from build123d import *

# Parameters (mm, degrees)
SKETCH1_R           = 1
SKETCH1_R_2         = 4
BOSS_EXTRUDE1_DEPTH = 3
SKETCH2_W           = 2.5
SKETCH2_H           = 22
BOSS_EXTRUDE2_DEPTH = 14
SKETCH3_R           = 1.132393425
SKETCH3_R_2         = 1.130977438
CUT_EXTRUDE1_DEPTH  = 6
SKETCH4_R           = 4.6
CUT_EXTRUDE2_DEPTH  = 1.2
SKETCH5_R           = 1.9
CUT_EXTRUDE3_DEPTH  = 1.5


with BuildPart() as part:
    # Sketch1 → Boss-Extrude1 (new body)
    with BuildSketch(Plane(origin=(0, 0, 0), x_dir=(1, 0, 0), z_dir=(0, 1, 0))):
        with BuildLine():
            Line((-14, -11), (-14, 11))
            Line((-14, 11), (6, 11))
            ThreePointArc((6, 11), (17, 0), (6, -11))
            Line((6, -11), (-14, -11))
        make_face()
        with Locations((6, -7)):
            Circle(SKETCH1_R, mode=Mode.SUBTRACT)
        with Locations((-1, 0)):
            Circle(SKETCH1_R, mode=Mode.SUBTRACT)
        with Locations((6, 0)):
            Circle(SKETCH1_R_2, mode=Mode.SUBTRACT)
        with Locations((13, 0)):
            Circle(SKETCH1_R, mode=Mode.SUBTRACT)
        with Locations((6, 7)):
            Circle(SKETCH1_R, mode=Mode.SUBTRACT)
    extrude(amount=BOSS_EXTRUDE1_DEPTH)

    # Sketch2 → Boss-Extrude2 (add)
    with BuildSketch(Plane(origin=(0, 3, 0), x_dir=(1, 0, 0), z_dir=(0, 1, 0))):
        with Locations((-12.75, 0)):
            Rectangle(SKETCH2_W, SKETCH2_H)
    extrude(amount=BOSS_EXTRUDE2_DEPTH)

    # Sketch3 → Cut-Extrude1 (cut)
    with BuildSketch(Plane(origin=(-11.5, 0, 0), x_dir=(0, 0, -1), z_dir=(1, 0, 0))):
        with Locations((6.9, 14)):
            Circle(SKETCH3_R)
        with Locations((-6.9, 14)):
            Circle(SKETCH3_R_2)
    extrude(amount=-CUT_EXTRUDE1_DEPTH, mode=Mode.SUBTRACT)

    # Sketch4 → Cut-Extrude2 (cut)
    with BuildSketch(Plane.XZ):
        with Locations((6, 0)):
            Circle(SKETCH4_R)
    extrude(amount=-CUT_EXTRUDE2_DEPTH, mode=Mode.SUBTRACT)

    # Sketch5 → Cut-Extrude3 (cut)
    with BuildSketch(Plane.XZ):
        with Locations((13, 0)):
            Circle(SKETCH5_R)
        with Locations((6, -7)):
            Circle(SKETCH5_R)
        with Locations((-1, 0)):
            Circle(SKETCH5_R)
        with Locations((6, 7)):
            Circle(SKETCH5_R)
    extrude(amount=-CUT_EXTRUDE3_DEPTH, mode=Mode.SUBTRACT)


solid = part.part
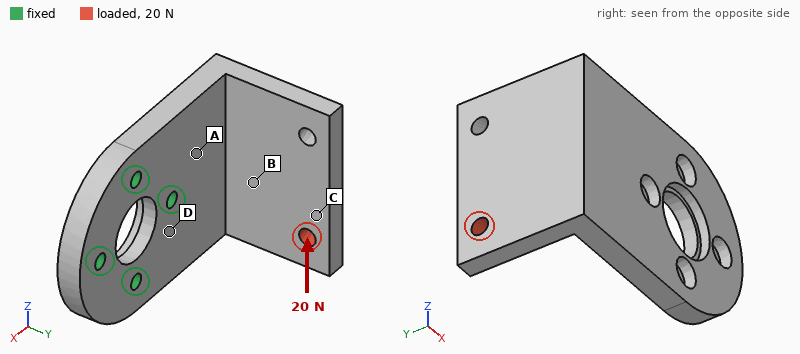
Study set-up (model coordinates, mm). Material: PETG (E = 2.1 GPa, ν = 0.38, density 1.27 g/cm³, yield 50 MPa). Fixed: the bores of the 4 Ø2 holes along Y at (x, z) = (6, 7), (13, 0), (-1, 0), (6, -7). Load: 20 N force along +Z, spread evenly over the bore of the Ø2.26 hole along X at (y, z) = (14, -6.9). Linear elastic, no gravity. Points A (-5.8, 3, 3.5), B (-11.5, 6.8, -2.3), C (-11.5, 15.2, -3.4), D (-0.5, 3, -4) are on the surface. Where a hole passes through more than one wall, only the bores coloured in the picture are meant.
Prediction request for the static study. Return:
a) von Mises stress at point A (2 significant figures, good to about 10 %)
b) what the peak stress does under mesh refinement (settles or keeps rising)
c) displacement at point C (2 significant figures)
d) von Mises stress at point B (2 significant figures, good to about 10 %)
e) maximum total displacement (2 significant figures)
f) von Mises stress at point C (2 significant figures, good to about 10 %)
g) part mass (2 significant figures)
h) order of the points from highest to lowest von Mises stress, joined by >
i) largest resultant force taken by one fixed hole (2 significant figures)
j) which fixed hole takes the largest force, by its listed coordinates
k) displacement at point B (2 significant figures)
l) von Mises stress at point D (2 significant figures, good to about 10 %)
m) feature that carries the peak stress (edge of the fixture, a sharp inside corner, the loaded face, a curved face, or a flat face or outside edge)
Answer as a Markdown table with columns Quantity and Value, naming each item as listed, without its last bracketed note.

| Quantity | Value |
|---|---|
| von Mises stress at point A | 6.4 MPa |
| what the peak stress does under mesh refinement | keeps rising |
| displacement at point C | 0.37 mm |
| von Mises stress at point B | 2.4 MPa |
| maximum total displacement | 0.49 mm |
| von Mises stress at point C | 1.3 MPa |
| part mass | 3.0 g |
| order of the points from highest to lowest von Mises stress, joined by > | A > D > B > C |
| largest resultant force taken by one fixed hole | 29 N |
| which fixed hole takes the largest force, by its listed coordinates | (-1, 0) |
| displacement at point B | 0.16 mm |
| von Mises stress at point D | 5.0 MPa |
| feature that carries the peak stress | edge of the fixture |
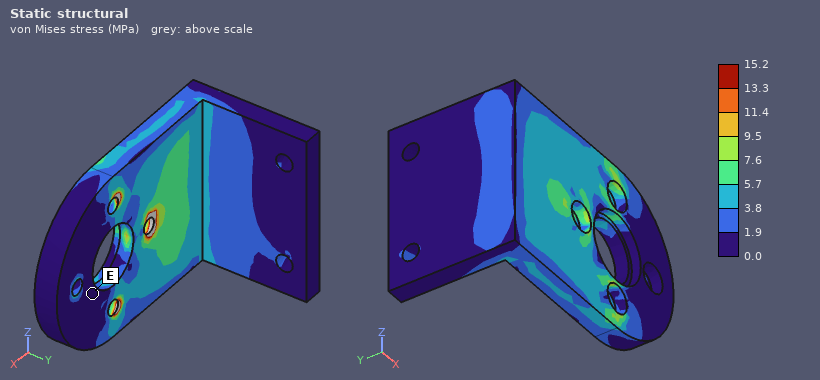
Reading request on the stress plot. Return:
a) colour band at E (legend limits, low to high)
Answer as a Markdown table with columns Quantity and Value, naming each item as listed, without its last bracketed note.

| Quantity | Value |
|---|---|
| colour band at E | 0.0 to 1.9 MPa |
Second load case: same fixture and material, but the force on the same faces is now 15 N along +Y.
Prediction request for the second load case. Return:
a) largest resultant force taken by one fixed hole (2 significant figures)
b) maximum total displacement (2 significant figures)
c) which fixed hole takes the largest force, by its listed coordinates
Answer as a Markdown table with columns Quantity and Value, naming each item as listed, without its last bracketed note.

| Quantity | Value |
|---|---|
| largest resultant force taken by one fixed hole | 34 N |
| maximum total displacement | 0.42 mm |
| which fixed hole takes the largest force, by its listed coordinates | (-1, 0) |
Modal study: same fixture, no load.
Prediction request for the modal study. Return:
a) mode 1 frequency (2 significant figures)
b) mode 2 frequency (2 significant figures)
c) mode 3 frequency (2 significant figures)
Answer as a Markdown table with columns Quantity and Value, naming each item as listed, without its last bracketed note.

| Quantity | Value |
|---|---|
| mode 1 frequency | 1000 Hz |
| mode 2 frequency | 1300 Hz |
| mode 3 frequency | 2400 Hz |
